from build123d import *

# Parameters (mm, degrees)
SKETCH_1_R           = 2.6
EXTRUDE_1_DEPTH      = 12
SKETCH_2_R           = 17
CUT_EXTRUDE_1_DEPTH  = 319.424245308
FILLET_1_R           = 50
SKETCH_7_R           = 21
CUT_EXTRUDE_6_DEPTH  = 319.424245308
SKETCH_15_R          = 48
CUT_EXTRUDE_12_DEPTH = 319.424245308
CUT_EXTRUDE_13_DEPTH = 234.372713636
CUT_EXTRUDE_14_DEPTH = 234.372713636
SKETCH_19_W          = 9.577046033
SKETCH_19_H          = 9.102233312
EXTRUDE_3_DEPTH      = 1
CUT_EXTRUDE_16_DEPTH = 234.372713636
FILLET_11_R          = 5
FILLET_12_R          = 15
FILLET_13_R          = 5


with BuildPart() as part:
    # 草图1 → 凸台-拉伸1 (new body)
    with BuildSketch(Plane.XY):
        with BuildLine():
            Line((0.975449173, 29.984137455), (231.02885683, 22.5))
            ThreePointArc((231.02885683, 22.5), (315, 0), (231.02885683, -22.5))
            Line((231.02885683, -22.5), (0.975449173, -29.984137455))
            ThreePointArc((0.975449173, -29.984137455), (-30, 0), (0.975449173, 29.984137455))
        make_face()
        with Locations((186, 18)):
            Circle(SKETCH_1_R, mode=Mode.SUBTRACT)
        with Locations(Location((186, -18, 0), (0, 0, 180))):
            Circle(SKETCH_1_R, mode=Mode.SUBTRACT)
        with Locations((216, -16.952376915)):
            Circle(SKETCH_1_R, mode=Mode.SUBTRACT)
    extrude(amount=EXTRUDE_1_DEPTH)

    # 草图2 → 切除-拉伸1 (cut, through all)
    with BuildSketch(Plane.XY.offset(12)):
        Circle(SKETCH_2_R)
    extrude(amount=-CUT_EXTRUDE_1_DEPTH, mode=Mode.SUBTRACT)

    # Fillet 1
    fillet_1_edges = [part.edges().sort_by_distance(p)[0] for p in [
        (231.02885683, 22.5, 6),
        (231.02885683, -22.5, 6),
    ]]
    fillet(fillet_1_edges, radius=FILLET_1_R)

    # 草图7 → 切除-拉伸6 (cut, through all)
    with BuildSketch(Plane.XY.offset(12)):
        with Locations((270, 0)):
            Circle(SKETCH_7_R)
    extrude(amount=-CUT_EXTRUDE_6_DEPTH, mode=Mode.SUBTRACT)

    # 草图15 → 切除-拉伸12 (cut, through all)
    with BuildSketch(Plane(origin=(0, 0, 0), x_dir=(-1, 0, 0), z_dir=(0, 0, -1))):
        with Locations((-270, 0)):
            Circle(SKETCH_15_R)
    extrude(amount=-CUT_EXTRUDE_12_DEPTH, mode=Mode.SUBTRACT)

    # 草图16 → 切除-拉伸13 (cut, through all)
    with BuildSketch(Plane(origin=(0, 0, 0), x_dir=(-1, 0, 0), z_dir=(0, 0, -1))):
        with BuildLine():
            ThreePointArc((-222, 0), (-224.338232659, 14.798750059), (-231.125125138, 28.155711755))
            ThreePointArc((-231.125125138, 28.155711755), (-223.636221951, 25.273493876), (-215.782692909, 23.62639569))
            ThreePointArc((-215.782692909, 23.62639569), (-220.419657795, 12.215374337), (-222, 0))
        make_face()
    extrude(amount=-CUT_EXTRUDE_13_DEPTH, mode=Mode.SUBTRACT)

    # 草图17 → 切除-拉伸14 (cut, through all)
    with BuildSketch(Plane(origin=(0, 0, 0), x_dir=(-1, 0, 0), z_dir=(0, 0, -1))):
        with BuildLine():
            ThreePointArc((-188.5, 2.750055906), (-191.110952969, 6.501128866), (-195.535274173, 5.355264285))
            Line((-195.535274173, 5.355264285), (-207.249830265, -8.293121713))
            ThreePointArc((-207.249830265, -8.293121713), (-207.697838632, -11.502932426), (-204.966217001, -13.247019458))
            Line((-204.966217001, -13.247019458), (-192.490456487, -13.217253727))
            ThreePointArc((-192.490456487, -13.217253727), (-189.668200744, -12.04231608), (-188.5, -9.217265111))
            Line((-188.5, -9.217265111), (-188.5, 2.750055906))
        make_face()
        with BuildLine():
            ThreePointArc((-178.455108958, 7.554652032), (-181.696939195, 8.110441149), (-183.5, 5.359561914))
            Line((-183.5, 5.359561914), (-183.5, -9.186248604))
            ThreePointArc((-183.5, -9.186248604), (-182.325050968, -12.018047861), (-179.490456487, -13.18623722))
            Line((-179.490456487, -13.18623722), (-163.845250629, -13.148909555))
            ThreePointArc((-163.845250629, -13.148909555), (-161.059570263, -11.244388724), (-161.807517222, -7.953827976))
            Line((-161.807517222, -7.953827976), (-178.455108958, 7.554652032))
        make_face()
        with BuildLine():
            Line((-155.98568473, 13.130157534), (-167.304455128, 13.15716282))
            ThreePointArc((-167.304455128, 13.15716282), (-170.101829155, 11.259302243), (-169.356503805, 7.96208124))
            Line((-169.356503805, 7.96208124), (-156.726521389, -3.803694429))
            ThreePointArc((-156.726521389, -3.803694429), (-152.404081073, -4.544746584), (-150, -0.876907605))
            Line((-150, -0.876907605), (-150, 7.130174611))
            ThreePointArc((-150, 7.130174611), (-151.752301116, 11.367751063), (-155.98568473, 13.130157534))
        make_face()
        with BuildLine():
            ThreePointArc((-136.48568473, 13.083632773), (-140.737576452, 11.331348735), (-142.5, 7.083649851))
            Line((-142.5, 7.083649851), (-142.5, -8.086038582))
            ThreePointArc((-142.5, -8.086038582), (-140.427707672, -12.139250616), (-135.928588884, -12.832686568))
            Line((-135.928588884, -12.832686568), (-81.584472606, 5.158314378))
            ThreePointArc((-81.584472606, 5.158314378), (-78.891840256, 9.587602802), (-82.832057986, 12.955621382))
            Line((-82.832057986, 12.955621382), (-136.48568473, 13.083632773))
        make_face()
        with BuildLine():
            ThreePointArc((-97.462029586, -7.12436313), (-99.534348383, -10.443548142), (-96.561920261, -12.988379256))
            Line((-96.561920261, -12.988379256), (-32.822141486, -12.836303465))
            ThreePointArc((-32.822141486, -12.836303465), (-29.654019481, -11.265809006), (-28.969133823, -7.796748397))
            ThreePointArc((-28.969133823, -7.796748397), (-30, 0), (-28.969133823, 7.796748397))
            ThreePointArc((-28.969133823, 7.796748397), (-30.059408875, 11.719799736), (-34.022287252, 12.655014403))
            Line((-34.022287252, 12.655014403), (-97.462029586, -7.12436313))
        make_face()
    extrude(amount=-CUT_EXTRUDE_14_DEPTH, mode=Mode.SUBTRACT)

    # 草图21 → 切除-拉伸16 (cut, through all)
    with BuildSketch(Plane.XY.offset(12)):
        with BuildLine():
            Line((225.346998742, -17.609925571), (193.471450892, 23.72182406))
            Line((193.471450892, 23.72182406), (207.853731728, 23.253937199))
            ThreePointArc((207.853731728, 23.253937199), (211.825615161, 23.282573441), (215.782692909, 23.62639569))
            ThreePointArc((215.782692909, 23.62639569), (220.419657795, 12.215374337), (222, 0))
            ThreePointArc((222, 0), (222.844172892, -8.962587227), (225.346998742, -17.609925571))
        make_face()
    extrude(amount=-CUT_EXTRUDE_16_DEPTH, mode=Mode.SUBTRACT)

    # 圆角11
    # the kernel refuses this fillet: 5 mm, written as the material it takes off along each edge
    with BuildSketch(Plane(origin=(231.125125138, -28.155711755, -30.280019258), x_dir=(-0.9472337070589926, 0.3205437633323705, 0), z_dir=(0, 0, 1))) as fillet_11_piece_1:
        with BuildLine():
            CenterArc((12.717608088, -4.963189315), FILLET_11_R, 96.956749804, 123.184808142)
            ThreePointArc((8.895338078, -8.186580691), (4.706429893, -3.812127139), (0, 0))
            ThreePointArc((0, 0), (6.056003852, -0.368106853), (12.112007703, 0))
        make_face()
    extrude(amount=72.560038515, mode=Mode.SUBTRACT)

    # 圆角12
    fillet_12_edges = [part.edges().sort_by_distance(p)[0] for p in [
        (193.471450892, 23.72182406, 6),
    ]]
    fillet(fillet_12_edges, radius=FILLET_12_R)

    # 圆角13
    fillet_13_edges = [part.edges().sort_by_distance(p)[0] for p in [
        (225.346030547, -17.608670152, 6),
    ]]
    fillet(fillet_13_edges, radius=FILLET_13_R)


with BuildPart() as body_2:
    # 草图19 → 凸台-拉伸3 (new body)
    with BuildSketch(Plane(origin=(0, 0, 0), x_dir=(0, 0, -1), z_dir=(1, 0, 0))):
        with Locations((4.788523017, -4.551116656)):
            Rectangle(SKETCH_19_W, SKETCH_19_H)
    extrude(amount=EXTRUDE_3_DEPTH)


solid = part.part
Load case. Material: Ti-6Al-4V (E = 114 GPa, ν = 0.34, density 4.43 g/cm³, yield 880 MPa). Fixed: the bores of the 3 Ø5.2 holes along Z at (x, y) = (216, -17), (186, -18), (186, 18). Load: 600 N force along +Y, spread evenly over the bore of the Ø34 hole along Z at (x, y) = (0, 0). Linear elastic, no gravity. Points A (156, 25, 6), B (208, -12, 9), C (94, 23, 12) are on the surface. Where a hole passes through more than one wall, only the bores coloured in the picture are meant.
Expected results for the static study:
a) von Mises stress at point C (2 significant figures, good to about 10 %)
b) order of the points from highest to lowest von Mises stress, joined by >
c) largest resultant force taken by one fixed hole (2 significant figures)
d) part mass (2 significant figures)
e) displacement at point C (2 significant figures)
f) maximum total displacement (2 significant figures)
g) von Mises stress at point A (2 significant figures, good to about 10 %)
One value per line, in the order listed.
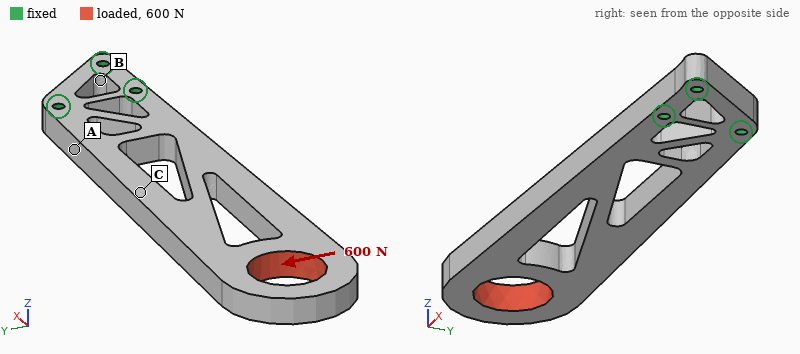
11 MPa
A > C > B
2.9 kN
460 g
0.054 mm
0.17 mm
19 MPa
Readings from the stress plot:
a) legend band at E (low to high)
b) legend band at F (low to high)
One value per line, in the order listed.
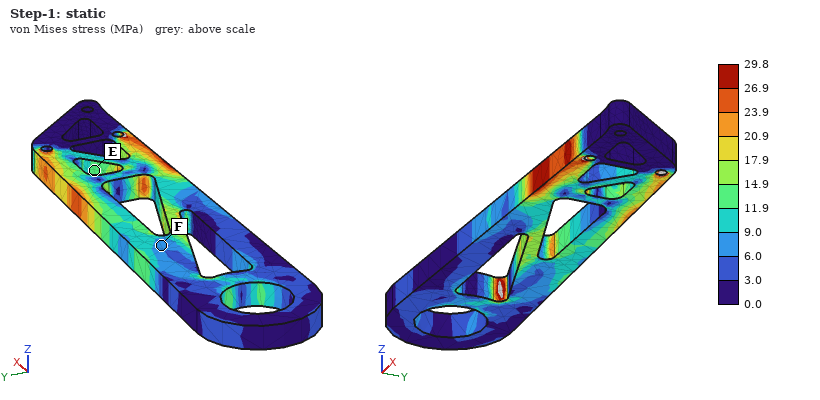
11.9 to 14.9 MPa
6.0 to 9.0 MPa
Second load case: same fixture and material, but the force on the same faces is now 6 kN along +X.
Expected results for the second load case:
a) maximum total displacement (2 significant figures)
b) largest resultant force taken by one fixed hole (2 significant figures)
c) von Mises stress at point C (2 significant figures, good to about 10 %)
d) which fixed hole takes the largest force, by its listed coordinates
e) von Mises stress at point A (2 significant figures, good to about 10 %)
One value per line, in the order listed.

34 µm
3.1 kN
16 MPa
(186, 18)
22 MPa
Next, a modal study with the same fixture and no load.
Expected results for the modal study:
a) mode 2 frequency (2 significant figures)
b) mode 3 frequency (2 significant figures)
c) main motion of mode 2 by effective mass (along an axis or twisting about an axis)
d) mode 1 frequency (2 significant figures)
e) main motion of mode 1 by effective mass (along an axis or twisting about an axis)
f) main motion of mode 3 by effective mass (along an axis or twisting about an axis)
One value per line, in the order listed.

790 Hz
1000 Hz
along Y
190 Hz
along Z
twisting about X
